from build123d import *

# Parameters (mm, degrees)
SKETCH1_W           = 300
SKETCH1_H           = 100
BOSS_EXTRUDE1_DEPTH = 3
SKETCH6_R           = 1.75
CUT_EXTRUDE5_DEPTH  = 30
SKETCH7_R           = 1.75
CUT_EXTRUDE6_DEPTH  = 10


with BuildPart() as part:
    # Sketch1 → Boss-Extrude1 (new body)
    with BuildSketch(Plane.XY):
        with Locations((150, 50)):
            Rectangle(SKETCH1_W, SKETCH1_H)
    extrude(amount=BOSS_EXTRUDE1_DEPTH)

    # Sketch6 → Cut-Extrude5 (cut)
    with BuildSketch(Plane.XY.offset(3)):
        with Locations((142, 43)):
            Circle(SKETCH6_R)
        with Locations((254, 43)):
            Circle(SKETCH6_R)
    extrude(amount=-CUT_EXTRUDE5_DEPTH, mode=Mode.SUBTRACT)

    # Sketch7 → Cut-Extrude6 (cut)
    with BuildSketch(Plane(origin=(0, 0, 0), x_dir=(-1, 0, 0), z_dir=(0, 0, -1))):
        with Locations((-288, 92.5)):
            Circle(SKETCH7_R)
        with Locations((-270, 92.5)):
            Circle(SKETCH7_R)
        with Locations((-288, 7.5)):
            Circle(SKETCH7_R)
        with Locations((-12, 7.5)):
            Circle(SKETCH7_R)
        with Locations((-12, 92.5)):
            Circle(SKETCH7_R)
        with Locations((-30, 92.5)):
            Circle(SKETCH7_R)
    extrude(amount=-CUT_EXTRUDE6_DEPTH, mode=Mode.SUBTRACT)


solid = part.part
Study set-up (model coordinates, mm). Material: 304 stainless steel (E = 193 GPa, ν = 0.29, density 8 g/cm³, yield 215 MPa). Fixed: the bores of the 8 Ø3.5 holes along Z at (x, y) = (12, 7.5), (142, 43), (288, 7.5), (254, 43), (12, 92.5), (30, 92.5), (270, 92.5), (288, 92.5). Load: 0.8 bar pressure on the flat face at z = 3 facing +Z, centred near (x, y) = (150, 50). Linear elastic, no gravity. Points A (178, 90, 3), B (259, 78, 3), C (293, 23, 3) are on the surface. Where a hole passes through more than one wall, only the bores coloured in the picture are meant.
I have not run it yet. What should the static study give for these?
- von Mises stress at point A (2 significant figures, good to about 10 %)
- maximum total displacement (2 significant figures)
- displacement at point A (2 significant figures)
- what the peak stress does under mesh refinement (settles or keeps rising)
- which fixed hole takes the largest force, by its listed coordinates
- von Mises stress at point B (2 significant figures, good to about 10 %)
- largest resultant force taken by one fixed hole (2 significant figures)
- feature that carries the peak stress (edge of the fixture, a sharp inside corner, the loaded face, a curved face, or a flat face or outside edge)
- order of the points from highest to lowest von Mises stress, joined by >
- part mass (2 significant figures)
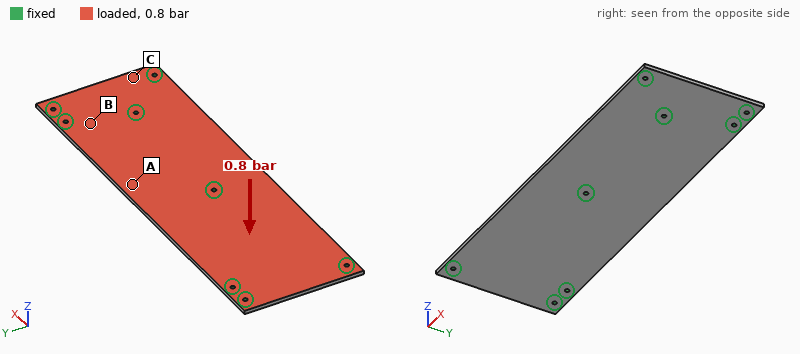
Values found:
23 MPa
0.26 mm
0.22 mm
keeps rising
(142, 43)
39 MPa
960 N
edge of the fixture
B > A > C
720 g
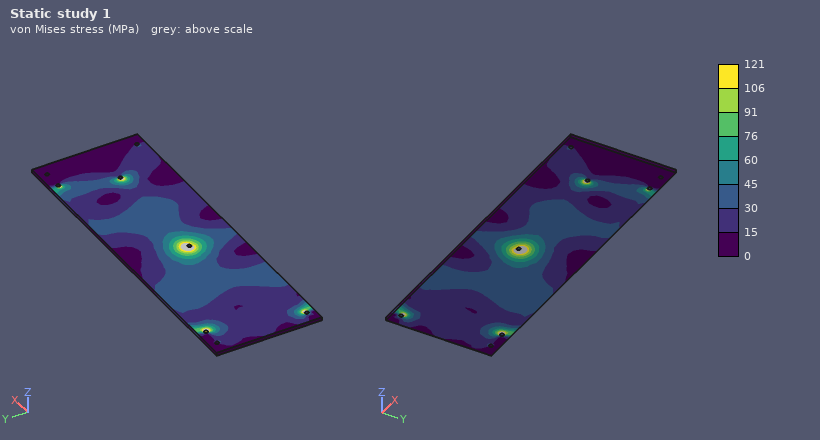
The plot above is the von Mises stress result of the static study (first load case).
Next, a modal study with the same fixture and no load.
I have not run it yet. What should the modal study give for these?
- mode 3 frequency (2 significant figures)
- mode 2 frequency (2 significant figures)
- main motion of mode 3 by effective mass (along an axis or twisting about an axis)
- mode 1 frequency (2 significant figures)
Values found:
860 Hz
770 Hz
along Z
640 Hz
